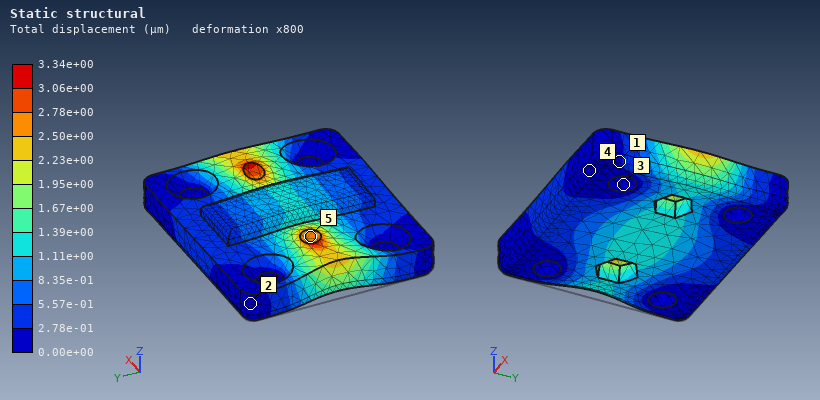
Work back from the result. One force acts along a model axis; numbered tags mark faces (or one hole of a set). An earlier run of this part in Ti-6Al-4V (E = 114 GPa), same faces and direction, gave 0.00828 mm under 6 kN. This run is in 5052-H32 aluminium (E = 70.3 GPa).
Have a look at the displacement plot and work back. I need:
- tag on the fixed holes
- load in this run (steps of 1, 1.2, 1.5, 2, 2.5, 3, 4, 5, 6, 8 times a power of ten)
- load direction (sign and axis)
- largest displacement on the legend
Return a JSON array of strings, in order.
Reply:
["3", "1.5 kN", "+X", "3.34e+00 µm"]
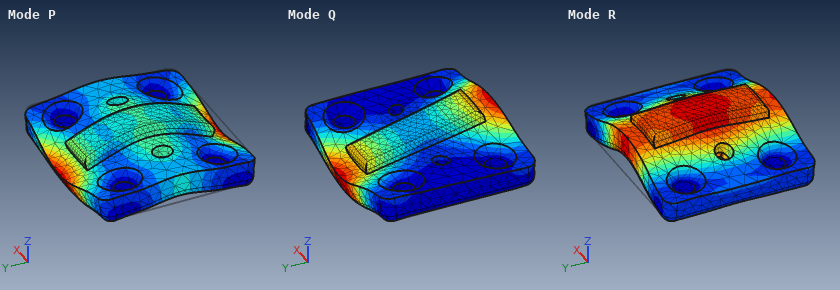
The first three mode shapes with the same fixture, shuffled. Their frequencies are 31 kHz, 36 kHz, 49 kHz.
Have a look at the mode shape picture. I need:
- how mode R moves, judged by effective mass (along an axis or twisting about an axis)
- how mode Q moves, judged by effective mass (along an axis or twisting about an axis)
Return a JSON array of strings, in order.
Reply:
["along Z", "twisting about X"]
